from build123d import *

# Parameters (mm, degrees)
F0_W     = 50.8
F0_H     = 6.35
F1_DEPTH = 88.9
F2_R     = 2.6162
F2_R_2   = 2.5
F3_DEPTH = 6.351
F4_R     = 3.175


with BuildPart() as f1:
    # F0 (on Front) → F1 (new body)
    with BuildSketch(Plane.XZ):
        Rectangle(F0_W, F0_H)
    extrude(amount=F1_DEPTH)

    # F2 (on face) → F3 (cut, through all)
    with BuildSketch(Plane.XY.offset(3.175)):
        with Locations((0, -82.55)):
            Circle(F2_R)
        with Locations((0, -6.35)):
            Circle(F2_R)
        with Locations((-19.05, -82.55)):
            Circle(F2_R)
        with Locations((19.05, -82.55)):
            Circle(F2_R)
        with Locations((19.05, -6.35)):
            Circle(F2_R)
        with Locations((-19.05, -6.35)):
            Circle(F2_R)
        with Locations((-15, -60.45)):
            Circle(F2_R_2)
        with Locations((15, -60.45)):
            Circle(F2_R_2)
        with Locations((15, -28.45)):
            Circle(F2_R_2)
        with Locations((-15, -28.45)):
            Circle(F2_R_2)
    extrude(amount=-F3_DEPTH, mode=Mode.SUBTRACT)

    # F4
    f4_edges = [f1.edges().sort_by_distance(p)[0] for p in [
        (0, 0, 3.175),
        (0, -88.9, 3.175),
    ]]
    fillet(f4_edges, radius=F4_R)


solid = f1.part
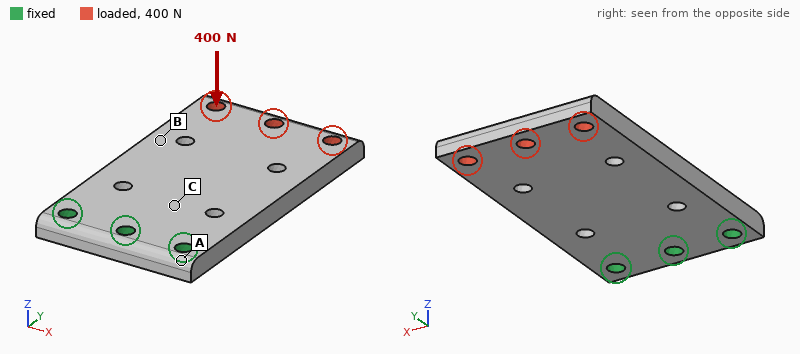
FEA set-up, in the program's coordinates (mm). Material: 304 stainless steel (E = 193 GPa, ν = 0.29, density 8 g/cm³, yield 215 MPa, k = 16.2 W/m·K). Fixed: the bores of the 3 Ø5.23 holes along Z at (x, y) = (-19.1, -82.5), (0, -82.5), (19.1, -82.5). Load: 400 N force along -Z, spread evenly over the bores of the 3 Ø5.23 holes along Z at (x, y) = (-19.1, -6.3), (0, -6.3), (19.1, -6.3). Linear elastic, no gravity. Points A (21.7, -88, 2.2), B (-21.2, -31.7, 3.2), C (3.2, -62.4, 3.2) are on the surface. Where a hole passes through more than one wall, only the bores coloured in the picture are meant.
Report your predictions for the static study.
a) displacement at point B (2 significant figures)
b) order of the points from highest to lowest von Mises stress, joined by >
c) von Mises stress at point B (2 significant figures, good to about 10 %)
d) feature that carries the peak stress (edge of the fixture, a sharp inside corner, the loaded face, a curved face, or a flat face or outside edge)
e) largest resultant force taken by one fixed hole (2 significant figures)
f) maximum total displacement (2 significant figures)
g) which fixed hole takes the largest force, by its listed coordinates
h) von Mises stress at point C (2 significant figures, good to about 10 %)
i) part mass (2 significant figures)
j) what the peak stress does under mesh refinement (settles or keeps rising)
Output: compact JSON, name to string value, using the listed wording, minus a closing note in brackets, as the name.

{"displacement at point B": "0.14 mm", "order of the points from highest to lowest von Mises stress, joined by >": "C > B > A", "von Mises stress at point B": "35 MPa", "feature that carries the peak stress": "edge of the fixture", "largest resultant force taken by one fixed hole": "340 N", "maximum total displacement": "0.32 mm", "which fixed hole takes the largest force, by its listed coordinates": "(0, -82.5)", "von Mises stress at point C": "67 MPa", "part mass": "220 g", "what the peak stress does under mesh refinement": "keeps rising"}
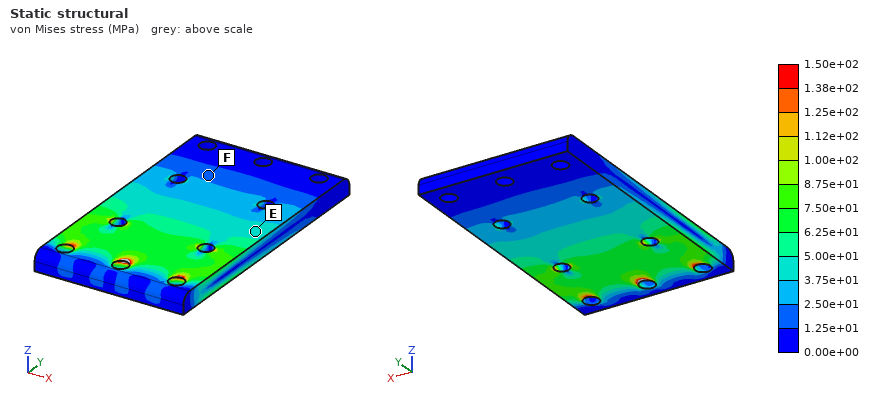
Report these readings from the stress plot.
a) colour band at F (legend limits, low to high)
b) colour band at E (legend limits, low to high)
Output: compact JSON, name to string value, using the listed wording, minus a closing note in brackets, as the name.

{"colour band at F": "1.25e+01 to 2.50e+01 MPa", "colour band at E": "3.75e+01 to 5.00e+01 MPa"}
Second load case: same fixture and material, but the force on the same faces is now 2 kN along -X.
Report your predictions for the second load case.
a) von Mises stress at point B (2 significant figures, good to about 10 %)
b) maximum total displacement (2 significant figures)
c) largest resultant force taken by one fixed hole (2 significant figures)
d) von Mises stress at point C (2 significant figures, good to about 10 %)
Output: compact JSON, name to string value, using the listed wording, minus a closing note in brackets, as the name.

{"von Mises stress at point B": "20 MPa", "maximum total displacement": "37 µm", "largest resultant force taken by one fixed hole": "3.8 kN", "von Mises stress at point C": "16 MPa"}
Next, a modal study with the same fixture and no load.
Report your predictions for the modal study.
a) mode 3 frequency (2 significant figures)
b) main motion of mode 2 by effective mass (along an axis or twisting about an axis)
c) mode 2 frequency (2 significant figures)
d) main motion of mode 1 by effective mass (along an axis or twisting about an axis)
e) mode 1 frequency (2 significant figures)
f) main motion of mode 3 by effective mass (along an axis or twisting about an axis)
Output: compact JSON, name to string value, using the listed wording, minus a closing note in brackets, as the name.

{"mode 3 frequency": "4700 Hz", "main motion of mode 2 by effective mass": "twisting about Y", "mode 2 frequency": "2600 Hz", "main motion of mode 1 by effective mass": "along Z", "mode 1 frequency": "770 Hz", "main motion of mode 3 by effective mass": "along Z"}
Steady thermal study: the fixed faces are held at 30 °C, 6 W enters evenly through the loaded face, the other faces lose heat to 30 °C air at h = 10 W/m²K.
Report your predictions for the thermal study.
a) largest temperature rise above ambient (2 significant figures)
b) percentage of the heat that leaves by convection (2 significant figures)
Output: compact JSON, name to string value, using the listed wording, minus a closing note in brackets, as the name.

{"largest temperature rise above ambient": "63 K", "percentage of the heat that leaves by convection": "48 %"}
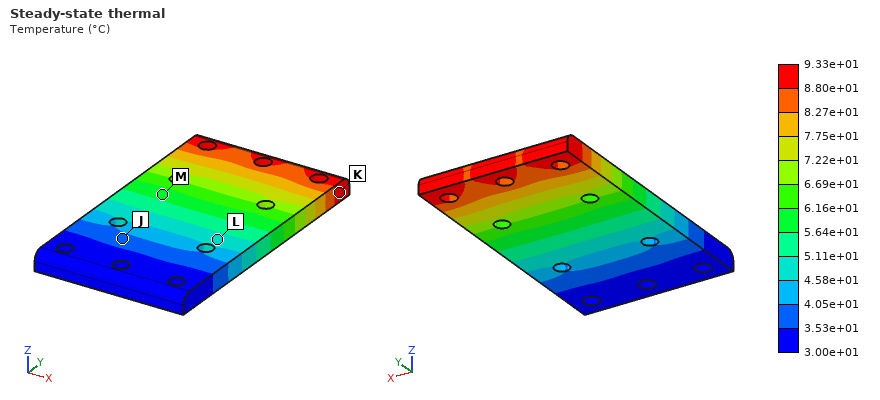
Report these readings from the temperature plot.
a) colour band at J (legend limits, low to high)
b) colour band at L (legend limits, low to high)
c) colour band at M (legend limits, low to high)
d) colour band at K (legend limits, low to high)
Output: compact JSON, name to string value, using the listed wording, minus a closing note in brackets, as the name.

{"colour band at J": "3.53e+01 to 4.05e+01 °C", "colour band at L": "4.58e+01 to 5.11e+01 °C", "colour band at M": "5.64e+01 to 6.16e+01 °C", "colour band at K": "8.80e+01 to 9.33e+01 °C"}
